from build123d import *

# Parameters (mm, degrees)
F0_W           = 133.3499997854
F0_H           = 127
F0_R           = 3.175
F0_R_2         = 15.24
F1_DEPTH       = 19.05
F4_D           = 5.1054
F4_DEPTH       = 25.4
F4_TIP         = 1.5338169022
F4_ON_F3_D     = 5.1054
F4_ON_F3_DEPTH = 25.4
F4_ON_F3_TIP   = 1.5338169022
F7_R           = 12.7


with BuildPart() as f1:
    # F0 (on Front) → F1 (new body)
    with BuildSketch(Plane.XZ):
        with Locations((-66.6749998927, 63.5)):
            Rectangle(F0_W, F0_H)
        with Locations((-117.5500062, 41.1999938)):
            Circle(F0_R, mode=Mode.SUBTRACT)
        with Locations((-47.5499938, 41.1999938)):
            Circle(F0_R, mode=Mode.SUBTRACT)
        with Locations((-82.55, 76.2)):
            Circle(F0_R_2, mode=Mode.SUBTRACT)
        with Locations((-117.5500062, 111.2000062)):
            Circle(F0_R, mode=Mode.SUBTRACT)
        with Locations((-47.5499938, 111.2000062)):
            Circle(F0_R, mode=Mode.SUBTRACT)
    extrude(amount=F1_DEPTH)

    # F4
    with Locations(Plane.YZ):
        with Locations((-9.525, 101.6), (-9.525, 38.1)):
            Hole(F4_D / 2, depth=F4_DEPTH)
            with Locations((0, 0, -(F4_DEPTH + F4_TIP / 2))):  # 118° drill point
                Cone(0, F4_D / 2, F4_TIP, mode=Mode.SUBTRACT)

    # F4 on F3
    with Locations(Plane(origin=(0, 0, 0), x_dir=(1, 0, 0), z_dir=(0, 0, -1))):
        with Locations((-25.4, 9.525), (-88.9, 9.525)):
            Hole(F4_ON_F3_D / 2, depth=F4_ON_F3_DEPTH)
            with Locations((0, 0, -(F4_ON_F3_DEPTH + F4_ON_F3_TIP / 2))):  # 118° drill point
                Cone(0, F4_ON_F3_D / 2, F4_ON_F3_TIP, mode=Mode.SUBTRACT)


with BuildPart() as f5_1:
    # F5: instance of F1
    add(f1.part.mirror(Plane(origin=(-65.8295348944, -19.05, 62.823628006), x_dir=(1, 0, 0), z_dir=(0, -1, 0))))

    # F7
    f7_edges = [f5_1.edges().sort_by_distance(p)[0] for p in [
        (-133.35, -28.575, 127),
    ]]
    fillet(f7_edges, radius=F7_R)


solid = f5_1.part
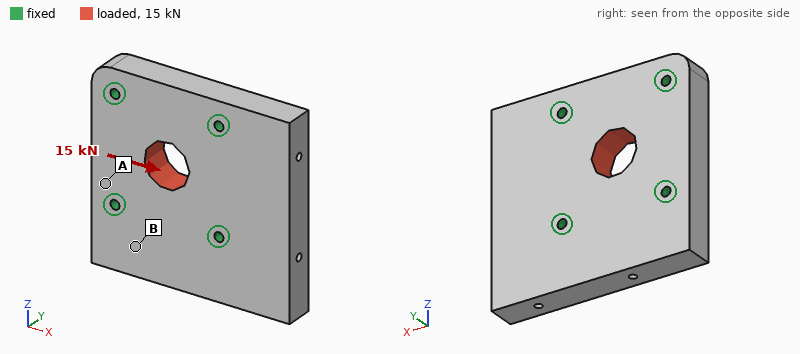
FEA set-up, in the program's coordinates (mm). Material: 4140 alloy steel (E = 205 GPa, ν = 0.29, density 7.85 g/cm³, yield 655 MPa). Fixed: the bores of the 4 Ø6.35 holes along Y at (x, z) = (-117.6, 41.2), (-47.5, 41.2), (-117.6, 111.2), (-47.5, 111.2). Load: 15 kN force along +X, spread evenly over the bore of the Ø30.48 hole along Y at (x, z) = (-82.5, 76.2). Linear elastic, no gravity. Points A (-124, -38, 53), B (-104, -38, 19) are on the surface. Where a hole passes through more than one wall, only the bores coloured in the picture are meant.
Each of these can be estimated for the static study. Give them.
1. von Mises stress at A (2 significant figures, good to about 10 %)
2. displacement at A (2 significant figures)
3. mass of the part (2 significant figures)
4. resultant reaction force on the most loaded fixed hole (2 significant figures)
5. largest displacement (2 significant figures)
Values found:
5.6 MPa
0.79 µm
2.4 kg
4.1 kN
2.2 µm
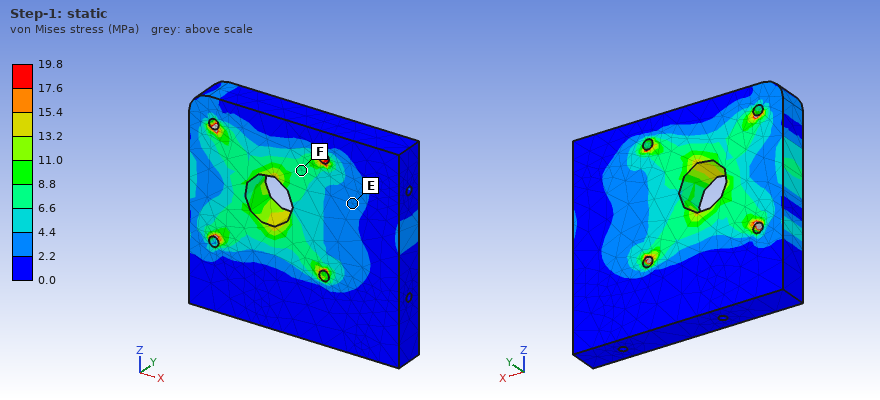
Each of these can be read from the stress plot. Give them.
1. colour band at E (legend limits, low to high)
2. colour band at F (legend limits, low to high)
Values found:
2.2 to 4.4 MPa
6.6 to 8.8 MPa
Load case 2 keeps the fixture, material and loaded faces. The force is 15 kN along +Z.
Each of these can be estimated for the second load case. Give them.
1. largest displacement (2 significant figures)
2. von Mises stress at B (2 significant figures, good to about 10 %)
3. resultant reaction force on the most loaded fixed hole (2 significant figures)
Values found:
2.2 µm
2.8 MPa
4.0 kN
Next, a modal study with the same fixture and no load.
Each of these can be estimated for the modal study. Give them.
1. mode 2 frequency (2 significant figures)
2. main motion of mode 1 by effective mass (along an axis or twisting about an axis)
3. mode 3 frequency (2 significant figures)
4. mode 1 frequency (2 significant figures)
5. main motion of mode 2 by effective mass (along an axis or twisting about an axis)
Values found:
5600 Hz
along Y
6900 Hz
4700 Hz
twisting about X
